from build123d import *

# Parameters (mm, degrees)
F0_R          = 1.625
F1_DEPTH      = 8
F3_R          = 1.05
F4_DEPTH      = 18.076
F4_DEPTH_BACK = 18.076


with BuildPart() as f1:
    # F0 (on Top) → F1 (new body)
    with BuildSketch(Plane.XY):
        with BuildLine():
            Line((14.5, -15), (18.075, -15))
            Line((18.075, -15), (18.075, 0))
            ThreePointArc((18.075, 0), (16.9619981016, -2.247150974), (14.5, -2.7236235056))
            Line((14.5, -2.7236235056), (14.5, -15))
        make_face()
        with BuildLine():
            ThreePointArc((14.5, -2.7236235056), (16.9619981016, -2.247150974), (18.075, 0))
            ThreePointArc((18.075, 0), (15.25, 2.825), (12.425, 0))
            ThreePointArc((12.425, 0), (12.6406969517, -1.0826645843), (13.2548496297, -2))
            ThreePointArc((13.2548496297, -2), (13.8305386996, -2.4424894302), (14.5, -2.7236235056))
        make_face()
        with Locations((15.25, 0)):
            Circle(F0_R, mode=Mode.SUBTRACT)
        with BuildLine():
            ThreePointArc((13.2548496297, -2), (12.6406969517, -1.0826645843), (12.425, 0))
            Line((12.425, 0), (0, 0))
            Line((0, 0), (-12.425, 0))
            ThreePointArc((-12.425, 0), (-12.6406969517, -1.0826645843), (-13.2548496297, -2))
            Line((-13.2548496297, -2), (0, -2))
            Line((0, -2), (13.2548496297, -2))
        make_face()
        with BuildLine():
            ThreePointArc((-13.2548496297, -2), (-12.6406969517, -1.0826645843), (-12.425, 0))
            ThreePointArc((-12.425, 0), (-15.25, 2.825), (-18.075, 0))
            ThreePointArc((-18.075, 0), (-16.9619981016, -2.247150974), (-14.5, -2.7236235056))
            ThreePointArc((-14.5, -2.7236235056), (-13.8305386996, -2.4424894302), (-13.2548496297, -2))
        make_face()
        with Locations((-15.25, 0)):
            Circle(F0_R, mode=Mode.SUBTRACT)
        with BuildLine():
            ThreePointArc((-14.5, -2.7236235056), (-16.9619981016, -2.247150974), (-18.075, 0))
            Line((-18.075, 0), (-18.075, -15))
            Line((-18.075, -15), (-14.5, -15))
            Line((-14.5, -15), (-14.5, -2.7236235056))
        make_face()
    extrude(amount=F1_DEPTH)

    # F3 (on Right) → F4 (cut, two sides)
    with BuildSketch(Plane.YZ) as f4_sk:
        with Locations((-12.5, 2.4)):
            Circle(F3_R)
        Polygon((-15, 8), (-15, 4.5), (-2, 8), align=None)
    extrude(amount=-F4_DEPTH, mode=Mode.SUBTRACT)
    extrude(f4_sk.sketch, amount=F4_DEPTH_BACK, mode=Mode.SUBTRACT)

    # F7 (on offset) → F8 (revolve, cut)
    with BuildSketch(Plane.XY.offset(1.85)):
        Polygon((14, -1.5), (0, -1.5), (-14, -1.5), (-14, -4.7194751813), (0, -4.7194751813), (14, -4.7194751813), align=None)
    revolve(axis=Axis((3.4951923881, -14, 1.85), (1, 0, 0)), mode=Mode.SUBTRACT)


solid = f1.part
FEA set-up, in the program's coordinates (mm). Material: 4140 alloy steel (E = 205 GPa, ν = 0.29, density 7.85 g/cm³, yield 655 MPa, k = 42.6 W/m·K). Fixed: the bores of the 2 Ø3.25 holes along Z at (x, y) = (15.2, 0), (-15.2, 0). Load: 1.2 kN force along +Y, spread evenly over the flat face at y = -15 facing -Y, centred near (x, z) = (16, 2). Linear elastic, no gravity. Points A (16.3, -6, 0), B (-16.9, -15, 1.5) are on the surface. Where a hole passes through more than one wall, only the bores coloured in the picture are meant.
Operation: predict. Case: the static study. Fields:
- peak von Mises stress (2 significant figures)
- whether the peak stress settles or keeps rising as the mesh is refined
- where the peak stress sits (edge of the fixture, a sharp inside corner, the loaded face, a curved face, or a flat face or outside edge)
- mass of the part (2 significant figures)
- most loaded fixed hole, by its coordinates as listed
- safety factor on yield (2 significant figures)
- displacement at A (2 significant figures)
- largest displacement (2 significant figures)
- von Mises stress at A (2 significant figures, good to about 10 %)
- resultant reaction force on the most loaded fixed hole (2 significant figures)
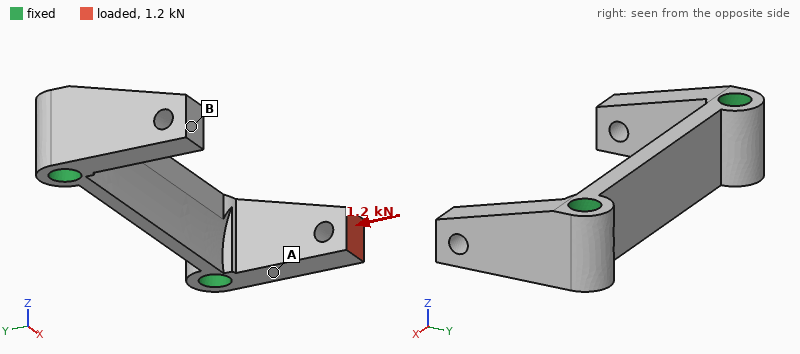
300 MPa
settles
a curved face
9.0 g
(15.2, 0)
2.2
2.8 µm
10 µm
99 MPa
1.2 kN
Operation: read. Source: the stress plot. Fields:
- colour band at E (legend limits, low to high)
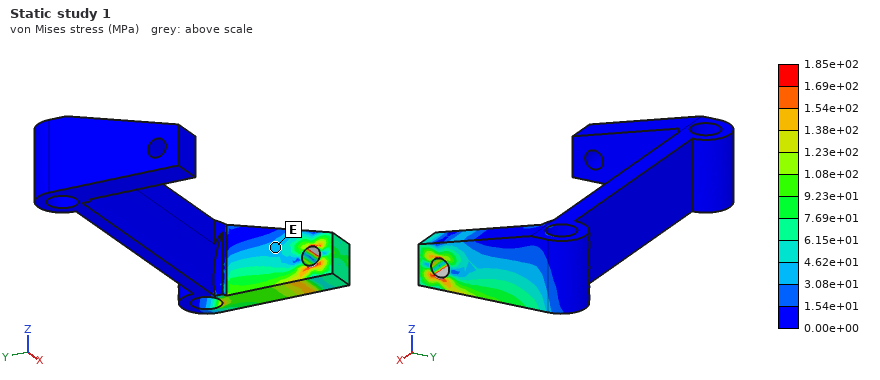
3.08e+01 to 4.62e+01 MPa
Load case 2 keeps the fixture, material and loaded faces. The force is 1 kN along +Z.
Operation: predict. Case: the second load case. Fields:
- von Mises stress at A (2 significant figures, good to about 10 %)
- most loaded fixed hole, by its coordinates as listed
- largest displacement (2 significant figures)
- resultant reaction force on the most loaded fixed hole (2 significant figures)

320 MPa
(15.2, 0)
57 µm
1.0 kN
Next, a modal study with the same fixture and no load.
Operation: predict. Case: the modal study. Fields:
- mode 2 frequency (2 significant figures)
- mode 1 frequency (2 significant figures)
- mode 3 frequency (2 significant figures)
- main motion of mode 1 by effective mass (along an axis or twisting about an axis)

18 kHz
13 kHz
18 kHz
along Y
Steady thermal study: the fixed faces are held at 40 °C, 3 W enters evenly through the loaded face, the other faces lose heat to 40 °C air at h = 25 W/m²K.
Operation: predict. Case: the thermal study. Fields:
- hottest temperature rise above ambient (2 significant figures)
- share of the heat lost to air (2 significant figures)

50 K
4.8 %
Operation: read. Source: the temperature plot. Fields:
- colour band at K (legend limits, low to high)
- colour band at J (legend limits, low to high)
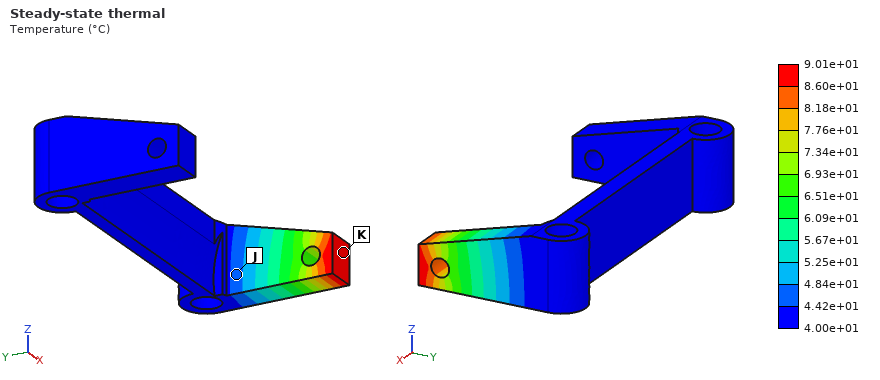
8.60e+01 to 9.01e+01 °C
4.42e+01 to 4.84e+01 °C
